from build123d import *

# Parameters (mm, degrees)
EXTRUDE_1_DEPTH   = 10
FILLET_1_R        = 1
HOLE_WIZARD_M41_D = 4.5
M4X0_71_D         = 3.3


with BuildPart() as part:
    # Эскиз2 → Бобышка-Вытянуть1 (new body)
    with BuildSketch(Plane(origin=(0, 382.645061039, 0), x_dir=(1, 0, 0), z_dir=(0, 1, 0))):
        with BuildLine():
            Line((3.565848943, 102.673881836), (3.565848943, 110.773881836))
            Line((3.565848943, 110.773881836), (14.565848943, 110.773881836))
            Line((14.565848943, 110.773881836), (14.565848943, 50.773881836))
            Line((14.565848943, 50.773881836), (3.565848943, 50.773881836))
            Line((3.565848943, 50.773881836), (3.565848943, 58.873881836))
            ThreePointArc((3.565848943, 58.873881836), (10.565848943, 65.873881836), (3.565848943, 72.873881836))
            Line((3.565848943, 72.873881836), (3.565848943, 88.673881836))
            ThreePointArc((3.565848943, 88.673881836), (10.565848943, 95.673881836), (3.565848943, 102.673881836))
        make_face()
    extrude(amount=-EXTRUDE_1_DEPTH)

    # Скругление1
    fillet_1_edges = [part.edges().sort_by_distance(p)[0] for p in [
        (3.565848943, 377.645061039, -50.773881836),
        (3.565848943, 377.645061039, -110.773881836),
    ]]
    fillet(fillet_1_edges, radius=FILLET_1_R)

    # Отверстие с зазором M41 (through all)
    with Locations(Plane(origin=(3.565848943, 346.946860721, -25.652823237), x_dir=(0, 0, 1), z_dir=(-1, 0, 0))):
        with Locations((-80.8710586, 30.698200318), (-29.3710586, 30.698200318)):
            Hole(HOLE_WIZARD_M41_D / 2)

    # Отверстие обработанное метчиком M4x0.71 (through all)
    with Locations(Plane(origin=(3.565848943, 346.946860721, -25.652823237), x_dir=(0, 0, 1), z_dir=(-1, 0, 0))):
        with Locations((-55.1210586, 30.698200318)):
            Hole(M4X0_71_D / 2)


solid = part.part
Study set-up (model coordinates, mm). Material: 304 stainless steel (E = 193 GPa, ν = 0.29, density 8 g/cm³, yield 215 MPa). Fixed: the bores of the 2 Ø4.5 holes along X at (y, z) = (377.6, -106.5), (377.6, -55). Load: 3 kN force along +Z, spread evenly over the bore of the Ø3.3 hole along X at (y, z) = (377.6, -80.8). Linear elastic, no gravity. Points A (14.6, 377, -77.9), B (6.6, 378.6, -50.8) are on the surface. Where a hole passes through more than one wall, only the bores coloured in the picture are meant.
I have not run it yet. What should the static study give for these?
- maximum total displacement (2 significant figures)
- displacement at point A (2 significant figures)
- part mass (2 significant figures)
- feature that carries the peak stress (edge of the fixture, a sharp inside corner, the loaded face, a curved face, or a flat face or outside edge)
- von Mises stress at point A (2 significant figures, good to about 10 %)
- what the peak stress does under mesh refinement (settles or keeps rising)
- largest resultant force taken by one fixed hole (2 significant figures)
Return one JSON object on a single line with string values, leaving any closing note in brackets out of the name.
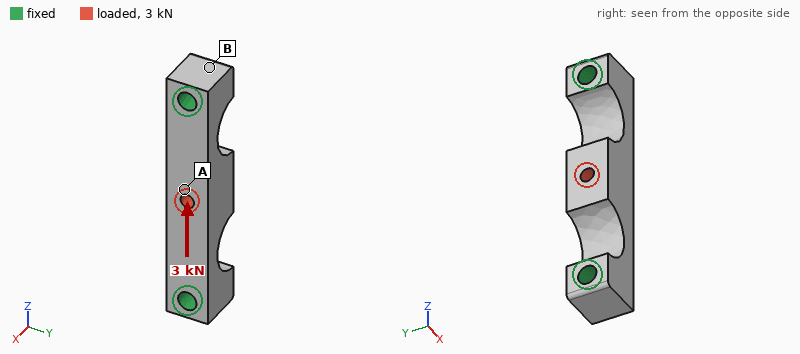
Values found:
{"maximum total displacement": "6.6 µm", "displacement at point A": "3.0 µm", "part mass": "37 g", "feature that carries the peak stress": "edge of the fixture", "von Mises stress at point A": "25 MPa", "what the peak stress does under mesh refinement": "keeps rising", "largest resultant force taken by one fixed hole": "1.5 kN"}
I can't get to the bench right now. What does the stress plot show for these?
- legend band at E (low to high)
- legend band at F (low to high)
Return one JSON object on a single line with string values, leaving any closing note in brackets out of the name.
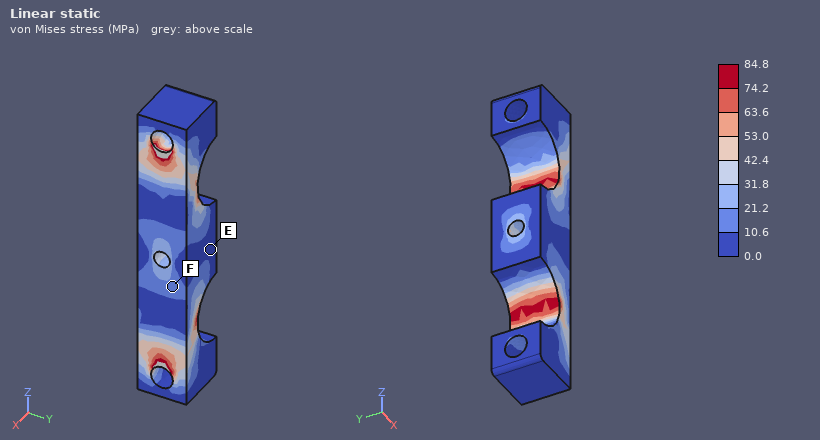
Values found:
{"legend band at E": "0.0 to 10.6 MPa", "legend band at F": "10.6 to 21.2 MPa"}
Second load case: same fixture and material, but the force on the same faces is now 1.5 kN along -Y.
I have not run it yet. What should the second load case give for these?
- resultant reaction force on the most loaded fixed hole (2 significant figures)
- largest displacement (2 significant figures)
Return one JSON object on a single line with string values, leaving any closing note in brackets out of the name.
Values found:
{"resultant reaction force on the most loaded fixed hole": "750 N", "largest displacement": "31 µm"}
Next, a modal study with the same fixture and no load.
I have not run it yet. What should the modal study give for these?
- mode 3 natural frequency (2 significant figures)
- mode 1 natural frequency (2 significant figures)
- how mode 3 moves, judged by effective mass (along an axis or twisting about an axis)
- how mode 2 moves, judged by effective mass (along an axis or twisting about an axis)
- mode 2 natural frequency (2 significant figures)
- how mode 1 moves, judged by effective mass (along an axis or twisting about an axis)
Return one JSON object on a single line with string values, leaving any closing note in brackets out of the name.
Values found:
{"mode 3 natural frequency": "20 kHz", "mode 1 natural frequency": "10 kHz", "how mode 3 moves, judged by effective mass": "along Y", "how mode 2 moves, judged by effective mass": "along X", "mode 2 natural frequency": "12 kHz", "how mode 1 moves, judged by effective mass": "along Y"}
